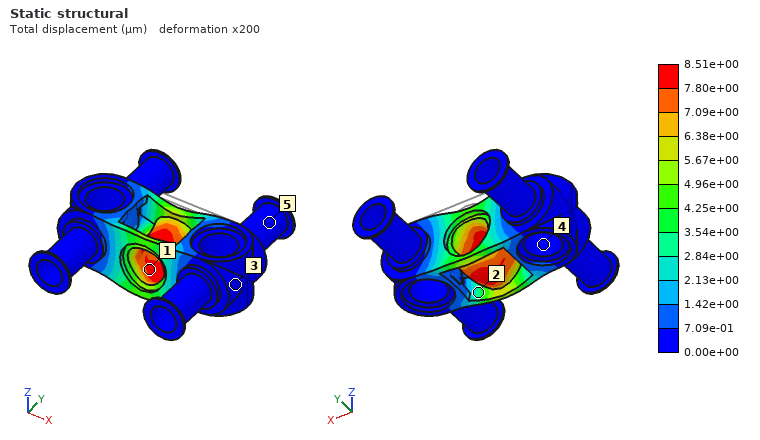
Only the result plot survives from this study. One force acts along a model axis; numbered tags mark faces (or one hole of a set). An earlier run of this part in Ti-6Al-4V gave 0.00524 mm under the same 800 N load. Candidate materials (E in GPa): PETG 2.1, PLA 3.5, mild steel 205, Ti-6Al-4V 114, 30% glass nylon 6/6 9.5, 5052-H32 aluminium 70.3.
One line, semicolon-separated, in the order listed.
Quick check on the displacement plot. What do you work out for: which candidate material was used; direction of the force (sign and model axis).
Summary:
5052-H32 aluminium; -Z
